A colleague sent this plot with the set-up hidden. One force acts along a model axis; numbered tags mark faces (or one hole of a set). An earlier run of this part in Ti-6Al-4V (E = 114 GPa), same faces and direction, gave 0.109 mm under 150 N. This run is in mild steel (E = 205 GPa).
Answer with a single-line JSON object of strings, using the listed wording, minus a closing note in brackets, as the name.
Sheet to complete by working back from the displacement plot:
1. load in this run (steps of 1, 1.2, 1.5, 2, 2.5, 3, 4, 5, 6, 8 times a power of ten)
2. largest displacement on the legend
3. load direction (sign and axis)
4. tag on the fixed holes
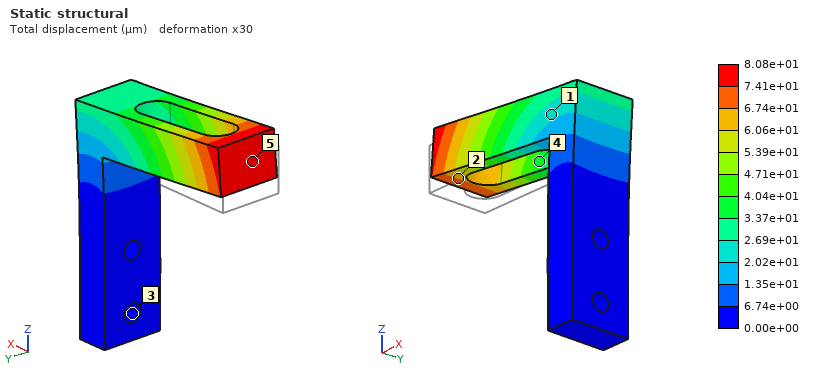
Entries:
{"load in this run": "200 N", "largest displacement on the legend": "8.08e+01 µm", "load direction": "+Z", "tag on the fixed holes": "3"}
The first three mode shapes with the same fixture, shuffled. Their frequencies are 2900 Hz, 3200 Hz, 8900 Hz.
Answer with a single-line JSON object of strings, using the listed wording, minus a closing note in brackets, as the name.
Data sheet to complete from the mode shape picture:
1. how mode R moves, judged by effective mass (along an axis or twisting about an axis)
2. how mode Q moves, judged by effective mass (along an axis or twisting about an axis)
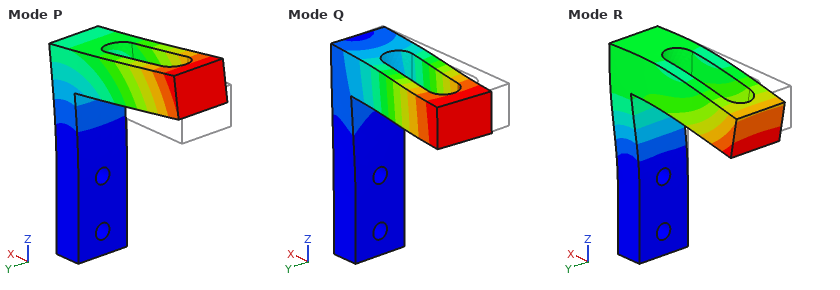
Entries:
{"how mode R moves, judged by effective mass": "along X", "how mode Q moves, judged by effective mass": "along Y"}
